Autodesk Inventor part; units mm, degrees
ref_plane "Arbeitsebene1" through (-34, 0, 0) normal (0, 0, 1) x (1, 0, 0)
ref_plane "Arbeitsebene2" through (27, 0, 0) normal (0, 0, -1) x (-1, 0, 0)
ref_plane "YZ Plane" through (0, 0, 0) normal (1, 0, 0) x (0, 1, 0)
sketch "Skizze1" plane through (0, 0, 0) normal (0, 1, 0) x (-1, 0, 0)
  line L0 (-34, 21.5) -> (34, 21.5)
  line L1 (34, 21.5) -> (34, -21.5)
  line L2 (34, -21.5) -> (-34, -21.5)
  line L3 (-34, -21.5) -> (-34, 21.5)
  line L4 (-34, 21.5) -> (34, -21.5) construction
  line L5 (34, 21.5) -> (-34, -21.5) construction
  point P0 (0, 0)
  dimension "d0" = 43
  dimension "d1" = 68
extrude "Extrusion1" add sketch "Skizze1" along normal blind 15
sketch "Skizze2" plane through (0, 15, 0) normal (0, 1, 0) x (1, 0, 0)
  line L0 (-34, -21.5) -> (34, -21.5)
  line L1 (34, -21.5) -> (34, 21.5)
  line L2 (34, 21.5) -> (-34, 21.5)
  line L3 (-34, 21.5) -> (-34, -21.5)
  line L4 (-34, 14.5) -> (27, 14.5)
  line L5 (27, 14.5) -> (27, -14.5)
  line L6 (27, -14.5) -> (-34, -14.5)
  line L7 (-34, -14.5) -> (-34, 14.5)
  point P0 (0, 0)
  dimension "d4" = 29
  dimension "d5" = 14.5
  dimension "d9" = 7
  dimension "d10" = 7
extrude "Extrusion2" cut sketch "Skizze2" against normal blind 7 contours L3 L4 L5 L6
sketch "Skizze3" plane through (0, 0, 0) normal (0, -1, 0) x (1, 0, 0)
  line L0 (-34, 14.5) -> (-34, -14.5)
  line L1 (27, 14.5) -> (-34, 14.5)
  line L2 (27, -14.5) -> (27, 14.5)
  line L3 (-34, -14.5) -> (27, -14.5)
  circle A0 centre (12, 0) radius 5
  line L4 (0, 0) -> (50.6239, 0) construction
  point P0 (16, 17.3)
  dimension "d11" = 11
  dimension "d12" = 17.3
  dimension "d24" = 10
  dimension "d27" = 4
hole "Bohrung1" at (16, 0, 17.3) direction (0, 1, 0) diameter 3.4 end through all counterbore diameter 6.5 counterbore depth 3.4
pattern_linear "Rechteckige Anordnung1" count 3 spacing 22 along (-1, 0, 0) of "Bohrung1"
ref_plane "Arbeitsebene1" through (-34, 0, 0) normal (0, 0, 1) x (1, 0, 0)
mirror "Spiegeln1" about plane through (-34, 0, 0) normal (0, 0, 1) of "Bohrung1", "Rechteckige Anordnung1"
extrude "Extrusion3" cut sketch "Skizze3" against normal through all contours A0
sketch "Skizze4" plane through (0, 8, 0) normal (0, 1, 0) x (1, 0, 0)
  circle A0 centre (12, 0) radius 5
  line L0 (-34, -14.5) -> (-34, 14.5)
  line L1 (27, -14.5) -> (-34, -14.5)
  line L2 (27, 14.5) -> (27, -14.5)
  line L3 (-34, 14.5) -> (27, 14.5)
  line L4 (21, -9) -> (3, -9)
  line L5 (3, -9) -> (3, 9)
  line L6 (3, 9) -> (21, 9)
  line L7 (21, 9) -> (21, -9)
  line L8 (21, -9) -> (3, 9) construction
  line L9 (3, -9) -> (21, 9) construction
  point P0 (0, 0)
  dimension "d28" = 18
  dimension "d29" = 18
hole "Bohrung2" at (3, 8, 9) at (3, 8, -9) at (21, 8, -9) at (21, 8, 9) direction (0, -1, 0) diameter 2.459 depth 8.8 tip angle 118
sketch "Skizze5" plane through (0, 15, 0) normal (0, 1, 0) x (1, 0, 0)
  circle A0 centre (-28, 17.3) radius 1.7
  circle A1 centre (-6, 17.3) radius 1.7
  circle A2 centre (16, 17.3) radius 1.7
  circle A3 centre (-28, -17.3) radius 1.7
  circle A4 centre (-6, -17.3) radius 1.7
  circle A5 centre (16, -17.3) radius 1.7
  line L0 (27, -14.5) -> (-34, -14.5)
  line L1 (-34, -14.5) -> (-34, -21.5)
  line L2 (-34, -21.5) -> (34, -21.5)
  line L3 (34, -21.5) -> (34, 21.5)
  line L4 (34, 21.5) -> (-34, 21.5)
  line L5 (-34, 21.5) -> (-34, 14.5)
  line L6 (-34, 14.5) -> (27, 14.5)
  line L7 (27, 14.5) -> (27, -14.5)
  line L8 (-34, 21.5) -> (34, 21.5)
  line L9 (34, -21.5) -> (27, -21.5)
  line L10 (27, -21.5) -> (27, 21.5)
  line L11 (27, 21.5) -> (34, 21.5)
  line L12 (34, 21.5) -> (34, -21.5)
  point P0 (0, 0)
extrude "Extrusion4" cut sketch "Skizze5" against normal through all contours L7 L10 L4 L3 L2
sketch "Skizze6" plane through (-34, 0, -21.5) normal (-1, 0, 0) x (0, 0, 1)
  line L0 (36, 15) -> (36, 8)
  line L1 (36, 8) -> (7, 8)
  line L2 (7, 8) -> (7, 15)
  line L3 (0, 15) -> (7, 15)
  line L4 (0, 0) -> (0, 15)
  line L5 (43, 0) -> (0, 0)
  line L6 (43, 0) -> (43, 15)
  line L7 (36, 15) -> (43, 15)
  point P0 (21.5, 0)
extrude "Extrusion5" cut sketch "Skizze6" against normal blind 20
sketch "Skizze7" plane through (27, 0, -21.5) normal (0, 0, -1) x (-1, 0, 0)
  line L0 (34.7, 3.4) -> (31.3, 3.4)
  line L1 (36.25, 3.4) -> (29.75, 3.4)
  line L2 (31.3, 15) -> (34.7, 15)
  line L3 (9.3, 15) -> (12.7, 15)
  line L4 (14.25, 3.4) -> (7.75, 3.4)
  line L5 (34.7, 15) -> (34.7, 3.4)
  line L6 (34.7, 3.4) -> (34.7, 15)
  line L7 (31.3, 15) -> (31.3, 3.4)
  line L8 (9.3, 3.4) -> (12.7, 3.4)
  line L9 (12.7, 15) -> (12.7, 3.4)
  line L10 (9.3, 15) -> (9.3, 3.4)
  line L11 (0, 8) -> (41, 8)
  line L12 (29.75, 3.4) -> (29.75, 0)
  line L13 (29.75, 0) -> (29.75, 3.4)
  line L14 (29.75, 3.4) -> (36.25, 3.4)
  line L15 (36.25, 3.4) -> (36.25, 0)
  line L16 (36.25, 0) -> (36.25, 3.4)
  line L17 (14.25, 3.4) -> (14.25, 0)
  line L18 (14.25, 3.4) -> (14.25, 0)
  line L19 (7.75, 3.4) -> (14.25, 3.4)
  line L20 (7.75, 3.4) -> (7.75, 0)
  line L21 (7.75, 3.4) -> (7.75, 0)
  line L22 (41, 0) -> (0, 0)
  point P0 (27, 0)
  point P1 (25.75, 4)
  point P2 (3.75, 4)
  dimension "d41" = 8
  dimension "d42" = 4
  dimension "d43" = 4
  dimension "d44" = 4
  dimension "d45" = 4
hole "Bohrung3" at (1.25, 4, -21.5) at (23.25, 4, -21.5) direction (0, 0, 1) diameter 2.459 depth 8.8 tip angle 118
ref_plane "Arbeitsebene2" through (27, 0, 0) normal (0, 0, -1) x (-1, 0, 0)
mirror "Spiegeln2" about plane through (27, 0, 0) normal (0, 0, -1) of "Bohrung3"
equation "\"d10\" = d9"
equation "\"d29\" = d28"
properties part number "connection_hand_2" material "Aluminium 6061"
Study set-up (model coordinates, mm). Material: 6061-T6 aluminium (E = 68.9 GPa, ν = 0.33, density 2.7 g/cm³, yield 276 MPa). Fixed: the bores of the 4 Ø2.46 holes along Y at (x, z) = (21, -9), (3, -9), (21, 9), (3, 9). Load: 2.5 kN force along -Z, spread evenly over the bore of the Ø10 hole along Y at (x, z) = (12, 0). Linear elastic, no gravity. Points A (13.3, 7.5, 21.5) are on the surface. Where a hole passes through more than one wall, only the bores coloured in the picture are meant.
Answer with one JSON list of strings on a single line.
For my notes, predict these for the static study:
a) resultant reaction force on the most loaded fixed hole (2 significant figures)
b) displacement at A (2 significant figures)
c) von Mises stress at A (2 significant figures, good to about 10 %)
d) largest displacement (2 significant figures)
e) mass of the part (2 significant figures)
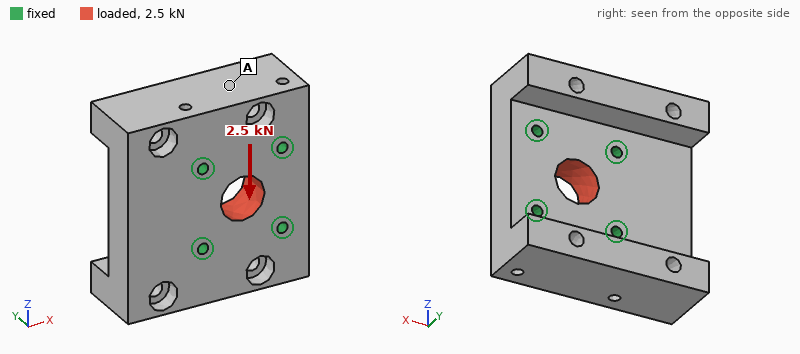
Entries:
["650 N", "0.72 µm", "3.6 MPa", "1.8 µm", "44 g"]
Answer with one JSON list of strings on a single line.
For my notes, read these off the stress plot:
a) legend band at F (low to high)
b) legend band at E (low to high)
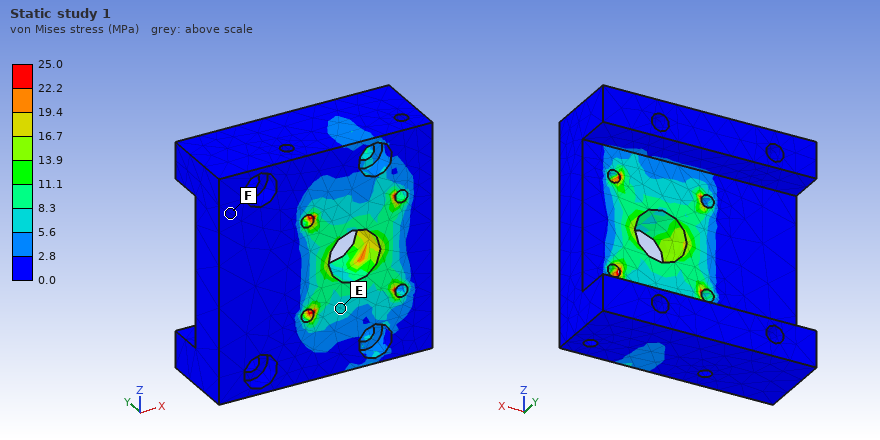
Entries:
["0.0 to 2.8 MPa", "5.6 to 8.3 MPa"]
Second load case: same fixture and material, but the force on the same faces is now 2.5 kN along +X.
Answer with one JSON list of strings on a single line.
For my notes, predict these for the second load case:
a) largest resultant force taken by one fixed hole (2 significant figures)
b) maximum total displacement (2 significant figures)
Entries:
["650 N", "2.1 µm"]
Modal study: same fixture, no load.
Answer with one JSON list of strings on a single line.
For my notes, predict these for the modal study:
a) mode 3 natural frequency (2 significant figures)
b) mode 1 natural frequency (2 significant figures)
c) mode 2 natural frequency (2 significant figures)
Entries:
["18 kHz", "14 kHz", "15 kHz"]
